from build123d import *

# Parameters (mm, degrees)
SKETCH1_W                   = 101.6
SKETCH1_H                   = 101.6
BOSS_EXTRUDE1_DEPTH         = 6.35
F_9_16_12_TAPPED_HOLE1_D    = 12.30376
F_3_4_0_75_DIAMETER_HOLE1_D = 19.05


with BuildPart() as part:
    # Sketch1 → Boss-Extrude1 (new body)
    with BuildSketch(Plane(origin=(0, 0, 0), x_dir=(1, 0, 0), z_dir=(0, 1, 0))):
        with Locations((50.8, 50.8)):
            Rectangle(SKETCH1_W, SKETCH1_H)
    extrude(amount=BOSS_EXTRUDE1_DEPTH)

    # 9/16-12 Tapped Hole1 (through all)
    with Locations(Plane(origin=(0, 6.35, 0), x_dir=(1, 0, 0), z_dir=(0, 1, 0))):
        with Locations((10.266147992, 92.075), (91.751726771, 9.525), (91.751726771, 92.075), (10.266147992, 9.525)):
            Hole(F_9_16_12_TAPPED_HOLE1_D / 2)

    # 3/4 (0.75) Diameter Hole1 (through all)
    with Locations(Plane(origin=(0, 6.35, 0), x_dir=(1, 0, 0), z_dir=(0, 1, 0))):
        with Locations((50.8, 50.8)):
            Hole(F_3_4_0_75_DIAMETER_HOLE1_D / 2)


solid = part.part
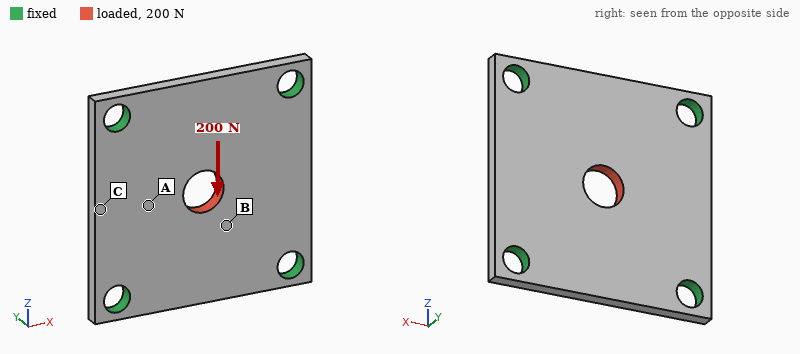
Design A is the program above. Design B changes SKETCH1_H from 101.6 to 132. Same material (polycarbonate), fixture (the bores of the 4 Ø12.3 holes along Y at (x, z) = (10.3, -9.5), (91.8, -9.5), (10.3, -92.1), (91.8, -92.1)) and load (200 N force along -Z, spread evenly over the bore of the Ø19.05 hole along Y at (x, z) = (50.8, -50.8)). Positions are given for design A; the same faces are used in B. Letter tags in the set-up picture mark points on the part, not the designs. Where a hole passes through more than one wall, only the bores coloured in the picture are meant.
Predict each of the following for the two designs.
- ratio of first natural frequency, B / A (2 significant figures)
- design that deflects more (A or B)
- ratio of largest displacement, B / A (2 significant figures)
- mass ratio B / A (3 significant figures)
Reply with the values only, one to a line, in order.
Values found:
1.0
A
0.90
1.32
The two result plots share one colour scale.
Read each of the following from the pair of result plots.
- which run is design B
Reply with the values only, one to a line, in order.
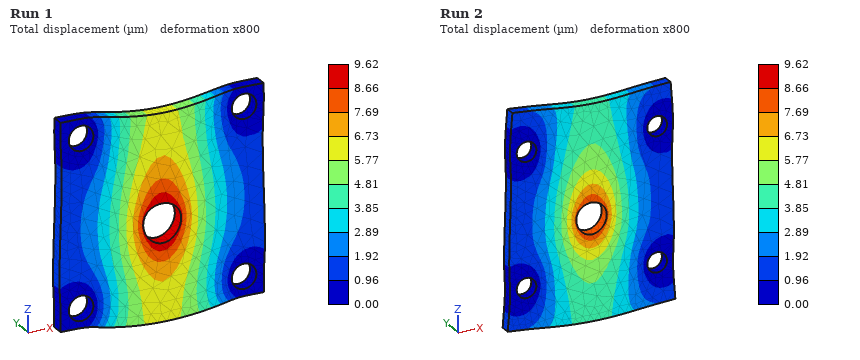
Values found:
Run 2
